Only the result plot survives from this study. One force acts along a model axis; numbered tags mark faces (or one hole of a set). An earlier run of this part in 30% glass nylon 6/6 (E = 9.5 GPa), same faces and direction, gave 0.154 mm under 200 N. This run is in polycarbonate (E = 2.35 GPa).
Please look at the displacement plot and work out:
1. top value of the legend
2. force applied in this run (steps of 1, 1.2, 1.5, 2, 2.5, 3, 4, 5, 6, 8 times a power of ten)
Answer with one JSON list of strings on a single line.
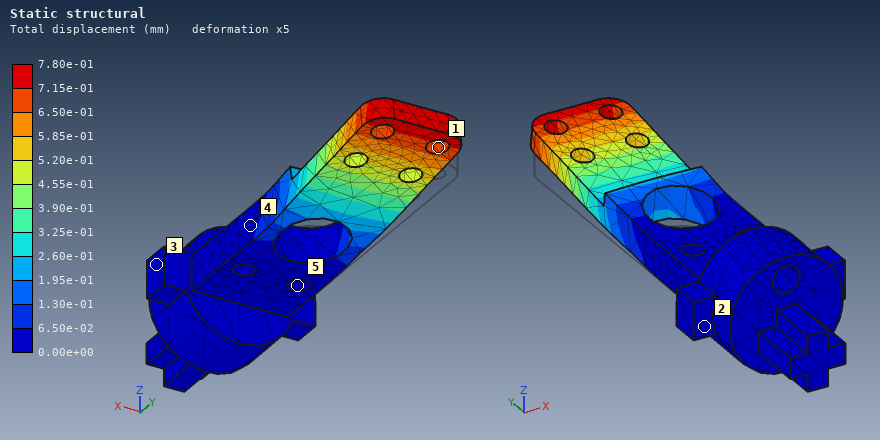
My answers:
["7.80e-01 mm", "250 N"]
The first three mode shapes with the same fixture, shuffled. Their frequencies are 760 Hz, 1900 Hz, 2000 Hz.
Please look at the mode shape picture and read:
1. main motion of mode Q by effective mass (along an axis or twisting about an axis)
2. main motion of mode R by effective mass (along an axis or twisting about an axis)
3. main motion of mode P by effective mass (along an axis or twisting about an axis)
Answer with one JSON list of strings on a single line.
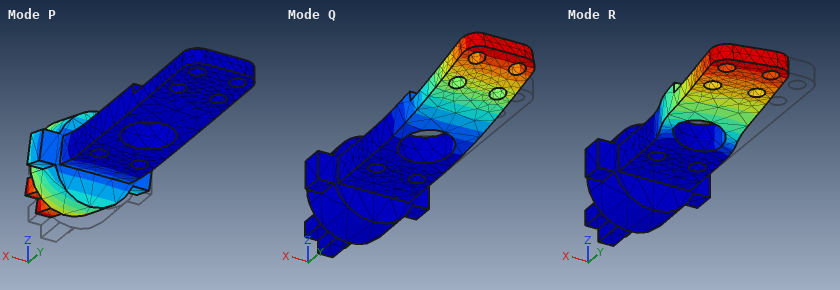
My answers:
["along Z", "along X", "along Z"]
